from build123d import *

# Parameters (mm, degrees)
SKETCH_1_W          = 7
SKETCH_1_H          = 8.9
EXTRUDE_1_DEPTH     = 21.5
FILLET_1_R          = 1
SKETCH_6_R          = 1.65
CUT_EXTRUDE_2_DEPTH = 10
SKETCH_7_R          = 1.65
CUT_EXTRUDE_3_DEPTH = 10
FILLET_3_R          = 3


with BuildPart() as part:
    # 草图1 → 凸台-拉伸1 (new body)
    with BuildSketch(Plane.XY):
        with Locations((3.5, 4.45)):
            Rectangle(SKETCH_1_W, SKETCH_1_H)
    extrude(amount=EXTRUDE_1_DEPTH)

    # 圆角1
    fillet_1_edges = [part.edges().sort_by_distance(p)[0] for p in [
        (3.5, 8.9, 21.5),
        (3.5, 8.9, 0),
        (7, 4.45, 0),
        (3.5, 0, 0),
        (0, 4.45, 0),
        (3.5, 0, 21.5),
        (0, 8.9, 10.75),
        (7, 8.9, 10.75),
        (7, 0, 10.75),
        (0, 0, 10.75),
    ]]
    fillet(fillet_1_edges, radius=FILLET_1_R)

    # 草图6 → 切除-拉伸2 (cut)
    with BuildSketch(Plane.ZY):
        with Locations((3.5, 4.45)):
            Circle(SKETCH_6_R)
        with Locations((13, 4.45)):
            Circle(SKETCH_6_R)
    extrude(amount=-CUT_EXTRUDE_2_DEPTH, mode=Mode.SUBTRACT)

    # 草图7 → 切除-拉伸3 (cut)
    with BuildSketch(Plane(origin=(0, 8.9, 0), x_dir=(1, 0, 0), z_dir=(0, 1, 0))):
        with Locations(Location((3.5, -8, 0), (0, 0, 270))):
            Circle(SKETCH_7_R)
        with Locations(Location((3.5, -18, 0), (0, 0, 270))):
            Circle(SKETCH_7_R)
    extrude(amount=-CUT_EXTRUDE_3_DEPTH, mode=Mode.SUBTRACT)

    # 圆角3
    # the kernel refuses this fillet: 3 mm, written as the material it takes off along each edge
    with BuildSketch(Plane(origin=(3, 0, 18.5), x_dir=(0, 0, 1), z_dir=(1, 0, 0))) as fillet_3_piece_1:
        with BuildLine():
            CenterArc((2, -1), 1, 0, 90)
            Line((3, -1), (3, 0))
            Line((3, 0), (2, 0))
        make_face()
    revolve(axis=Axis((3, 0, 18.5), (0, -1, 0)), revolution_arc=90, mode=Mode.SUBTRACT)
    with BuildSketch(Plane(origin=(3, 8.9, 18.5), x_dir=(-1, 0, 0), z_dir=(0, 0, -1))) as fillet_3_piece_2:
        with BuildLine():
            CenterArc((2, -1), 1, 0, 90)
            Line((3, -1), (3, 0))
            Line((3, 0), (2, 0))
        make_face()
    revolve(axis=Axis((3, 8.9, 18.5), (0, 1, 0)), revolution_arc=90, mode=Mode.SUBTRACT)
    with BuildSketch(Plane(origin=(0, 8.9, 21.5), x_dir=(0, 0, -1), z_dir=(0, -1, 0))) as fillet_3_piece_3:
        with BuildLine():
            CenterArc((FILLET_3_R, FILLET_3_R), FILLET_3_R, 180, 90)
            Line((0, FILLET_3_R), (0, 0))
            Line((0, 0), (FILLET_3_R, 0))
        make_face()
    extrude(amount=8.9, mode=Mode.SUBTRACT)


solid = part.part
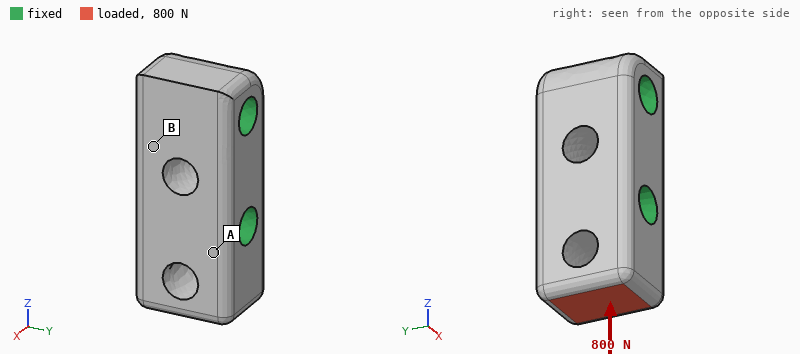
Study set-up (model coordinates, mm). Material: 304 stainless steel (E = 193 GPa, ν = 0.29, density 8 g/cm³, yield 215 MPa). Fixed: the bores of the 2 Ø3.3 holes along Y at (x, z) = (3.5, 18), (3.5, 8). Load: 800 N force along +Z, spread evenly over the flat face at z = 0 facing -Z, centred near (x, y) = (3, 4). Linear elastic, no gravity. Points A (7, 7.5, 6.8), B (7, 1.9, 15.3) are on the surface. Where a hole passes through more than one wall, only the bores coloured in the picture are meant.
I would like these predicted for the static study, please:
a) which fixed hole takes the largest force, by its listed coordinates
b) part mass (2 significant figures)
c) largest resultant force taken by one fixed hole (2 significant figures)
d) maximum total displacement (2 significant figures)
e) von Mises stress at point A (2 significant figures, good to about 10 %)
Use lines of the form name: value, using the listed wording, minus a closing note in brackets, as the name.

which fixed hole takes the largest force, by its listed coordinates: (3.5, 8)
part mass: 8.2 g
largest resultant force taken by one fixed hole: 780 N
maximum total displacement: 1.3 µm
von Mises stress at point A: 11 MPa
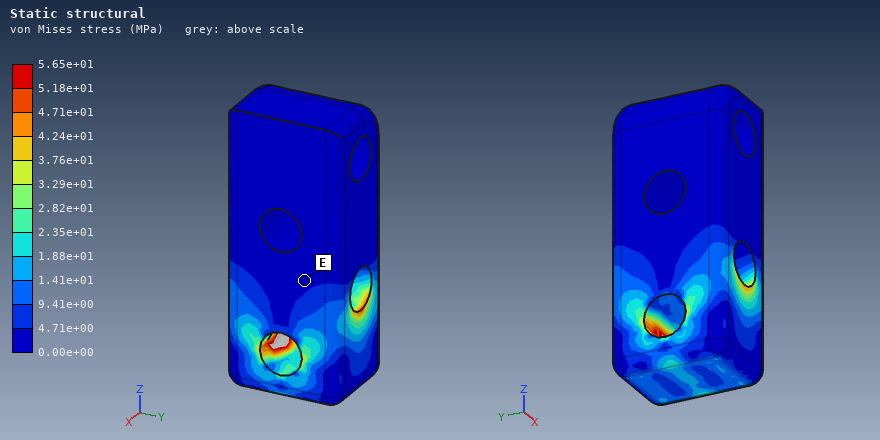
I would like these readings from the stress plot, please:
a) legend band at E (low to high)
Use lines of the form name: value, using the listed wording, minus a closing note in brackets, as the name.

legend band at E: 0.00e+00 to 4.71e+00 MPa
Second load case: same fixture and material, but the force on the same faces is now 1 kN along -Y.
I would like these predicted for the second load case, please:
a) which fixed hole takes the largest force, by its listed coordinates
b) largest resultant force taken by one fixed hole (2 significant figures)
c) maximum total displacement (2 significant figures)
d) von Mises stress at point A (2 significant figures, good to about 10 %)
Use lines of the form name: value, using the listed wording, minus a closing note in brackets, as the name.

which fixed hole takes the largest force, by its listed coordinates: (3.5, 8)
largest resultant force taken by one fixed hole: 1.0 kN
maximum total displacement: 5.9 µm
von Mises stress at point A: 23 MPa
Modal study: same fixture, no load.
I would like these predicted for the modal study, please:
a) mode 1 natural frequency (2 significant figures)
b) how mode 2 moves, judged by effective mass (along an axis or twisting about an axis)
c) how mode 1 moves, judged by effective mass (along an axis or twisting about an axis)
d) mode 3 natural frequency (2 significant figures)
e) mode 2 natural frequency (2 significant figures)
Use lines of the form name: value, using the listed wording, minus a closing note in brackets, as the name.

mode 1 natural frequency: 59 kHz
how mode 2 moves, judged by effective mass: along Y
how mode 1 moves, judged by effective mass: along X
mode 3 natural frequency: 88 kHz
mode 2 natural frequency: 67 kHz
